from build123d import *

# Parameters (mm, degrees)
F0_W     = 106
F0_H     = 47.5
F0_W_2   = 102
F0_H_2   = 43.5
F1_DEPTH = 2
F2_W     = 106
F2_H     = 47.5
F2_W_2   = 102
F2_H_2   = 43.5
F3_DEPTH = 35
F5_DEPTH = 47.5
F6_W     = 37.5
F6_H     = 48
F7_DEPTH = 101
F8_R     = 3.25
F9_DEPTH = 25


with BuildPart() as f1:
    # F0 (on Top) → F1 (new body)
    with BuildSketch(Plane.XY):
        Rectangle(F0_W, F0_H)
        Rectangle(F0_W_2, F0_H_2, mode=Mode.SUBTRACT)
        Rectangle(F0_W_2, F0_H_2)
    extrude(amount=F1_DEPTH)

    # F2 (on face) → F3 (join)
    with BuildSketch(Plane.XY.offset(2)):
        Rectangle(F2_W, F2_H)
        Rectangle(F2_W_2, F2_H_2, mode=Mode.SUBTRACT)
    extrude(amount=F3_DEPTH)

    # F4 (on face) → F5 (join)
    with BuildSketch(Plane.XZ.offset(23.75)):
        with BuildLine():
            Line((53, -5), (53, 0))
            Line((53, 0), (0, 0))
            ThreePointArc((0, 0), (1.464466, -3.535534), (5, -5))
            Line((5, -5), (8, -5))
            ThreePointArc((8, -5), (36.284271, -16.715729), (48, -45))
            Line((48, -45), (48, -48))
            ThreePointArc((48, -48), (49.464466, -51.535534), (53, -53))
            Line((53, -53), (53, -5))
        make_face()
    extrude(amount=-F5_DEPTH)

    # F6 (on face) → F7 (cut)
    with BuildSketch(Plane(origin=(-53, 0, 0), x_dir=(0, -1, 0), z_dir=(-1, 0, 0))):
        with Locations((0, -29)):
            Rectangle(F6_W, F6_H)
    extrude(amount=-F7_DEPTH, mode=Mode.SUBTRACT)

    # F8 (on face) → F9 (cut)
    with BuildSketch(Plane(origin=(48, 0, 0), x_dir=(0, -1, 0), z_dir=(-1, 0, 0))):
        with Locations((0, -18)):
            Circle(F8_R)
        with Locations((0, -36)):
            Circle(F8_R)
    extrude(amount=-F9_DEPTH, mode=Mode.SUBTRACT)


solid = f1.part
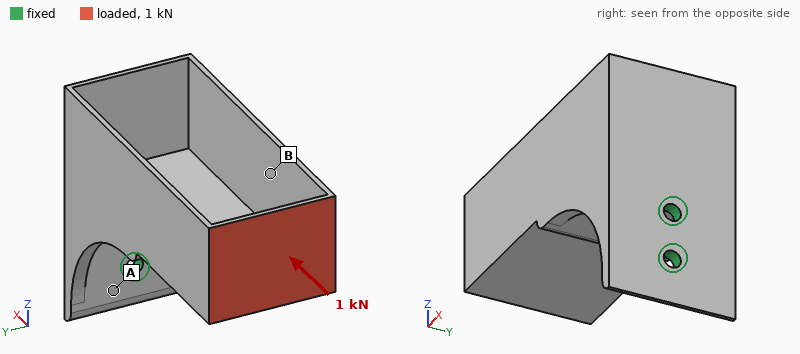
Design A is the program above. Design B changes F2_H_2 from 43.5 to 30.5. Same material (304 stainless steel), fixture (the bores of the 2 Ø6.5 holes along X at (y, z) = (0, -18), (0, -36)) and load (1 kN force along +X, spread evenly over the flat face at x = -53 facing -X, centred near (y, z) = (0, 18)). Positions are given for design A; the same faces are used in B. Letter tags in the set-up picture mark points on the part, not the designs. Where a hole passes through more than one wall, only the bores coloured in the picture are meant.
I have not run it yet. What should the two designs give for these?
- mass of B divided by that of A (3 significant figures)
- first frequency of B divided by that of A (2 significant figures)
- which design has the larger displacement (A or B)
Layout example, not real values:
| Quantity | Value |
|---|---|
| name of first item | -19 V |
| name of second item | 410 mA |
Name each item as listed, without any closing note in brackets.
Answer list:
| Quantity | Value |
|---|---|
| mass of B divided by that of A | 1.81 |
| first frequency of B divided by that of A | 0.67 |
| which design has the larger displacement | A |
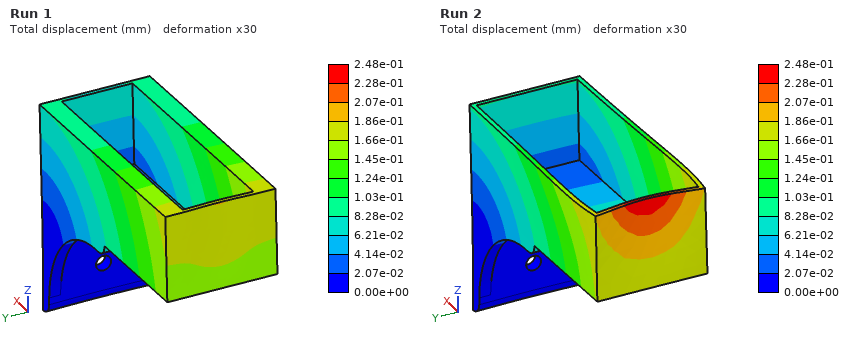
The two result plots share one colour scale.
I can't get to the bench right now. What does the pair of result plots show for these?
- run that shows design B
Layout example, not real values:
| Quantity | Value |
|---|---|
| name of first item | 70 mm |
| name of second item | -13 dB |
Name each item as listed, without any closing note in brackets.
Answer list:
| Quantity | Value |
|---|---|
| run that shows design B | Run 1 |
